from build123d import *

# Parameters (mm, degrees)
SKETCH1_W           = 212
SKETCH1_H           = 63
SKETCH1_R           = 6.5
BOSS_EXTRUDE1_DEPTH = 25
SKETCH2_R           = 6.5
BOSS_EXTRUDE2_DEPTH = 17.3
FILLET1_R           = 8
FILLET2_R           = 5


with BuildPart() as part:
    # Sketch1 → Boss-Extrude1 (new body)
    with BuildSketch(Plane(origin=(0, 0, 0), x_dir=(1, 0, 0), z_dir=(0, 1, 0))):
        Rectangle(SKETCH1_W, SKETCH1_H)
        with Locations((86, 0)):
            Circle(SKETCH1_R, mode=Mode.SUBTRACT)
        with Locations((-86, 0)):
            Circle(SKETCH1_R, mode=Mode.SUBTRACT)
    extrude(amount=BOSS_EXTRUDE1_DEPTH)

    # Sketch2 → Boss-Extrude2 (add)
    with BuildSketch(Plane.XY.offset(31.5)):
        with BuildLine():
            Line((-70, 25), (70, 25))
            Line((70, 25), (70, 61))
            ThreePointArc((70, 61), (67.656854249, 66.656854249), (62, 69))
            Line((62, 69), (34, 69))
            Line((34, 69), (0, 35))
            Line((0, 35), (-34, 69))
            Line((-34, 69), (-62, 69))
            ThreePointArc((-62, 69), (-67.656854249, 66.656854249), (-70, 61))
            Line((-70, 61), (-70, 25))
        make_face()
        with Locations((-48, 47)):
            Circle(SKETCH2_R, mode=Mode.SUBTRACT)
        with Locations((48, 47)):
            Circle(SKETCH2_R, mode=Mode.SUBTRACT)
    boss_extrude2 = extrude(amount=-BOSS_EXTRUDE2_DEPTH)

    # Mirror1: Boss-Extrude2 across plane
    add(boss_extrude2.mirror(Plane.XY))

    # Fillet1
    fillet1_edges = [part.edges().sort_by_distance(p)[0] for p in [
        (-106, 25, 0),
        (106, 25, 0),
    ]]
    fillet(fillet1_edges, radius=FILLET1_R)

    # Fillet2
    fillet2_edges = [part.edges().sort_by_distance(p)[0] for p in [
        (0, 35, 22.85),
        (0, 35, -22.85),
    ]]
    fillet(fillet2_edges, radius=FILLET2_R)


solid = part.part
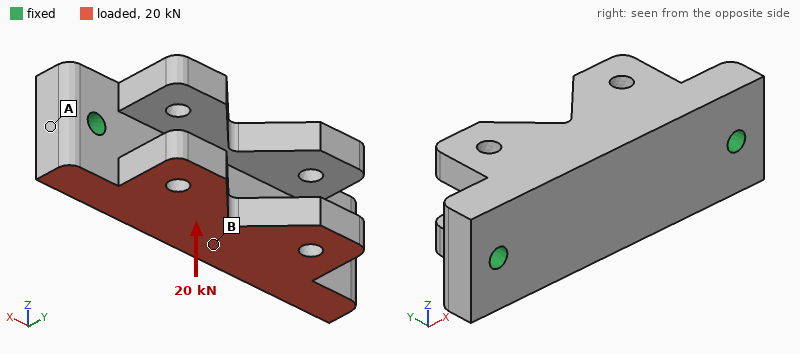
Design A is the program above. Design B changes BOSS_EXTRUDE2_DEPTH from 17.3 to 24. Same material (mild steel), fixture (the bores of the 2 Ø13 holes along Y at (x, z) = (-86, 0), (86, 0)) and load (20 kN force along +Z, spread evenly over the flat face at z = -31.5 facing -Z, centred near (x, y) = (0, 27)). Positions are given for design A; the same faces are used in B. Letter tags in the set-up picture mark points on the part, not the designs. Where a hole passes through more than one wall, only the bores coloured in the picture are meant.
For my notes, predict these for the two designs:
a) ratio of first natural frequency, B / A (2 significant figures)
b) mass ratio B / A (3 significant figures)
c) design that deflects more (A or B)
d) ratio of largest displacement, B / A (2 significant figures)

0.96
1.13
A
0.73
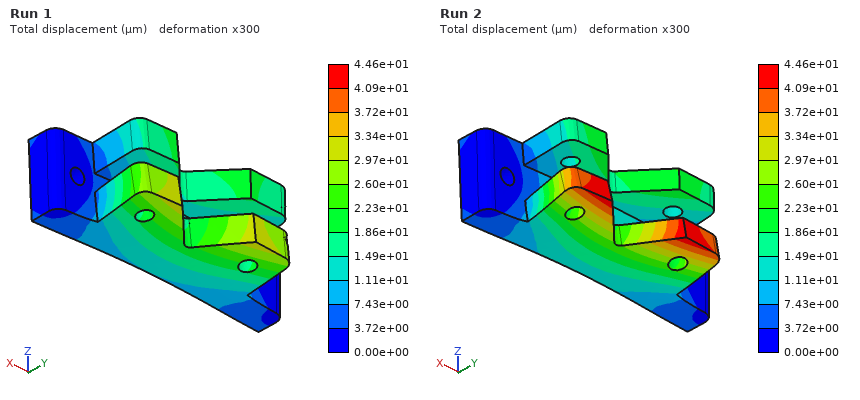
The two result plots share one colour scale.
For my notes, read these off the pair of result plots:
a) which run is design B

Run 1
